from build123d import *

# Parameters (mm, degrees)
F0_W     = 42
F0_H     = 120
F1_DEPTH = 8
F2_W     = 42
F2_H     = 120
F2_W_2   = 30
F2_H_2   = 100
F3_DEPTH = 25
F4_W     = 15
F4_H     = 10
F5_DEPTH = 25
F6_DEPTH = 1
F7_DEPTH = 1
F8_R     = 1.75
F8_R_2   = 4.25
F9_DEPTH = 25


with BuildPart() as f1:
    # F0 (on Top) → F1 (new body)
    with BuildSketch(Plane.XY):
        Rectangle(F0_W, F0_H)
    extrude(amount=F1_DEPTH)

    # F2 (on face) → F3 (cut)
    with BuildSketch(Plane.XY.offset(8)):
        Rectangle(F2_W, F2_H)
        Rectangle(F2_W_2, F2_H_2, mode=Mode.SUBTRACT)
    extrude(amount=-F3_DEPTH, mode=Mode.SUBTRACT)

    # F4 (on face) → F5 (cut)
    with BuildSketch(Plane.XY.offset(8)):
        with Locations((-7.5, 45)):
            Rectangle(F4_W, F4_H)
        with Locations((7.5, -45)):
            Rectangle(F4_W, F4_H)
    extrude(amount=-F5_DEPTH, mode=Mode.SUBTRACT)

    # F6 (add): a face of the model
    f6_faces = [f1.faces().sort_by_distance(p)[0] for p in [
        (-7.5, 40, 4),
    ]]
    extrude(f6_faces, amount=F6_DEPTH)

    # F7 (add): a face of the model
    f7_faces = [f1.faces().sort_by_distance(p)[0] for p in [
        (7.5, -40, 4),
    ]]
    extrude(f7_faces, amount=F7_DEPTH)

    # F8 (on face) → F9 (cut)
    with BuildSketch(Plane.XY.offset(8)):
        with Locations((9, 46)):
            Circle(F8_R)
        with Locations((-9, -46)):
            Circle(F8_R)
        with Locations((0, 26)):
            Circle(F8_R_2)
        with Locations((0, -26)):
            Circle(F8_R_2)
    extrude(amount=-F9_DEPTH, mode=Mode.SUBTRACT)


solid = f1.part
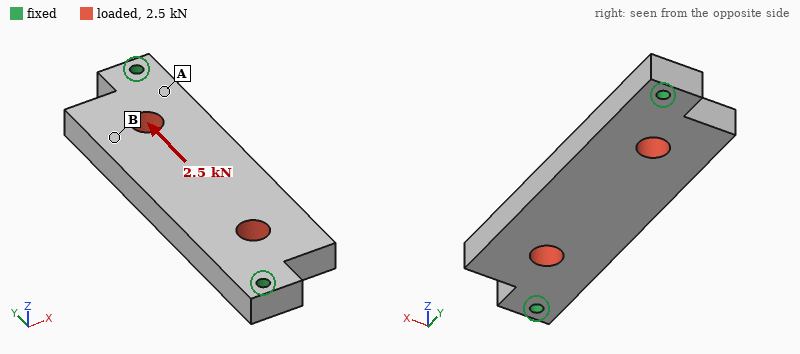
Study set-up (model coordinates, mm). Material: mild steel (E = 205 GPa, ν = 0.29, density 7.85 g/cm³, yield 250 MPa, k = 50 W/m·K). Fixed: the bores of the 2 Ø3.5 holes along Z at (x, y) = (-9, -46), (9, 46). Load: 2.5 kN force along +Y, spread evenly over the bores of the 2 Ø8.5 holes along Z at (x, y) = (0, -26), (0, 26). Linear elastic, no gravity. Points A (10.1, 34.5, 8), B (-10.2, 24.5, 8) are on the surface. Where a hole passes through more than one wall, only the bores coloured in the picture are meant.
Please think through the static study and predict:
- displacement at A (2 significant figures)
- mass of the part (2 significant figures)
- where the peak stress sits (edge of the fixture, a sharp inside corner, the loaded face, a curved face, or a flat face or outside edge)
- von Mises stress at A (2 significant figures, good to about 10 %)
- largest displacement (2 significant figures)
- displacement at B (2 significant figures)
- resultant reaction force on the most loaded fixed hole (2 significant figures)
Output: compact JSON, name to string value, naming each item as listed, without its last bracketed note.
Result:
{"displacement at A": "1.2 µm", "mass of the part": "160 g", "where the peak stress sits": "edge of the fixture", "von Mises stress at A": "11 MPa", "largest displacement": "3.3 µm", "displacement at B": "3.0 µm", "resultant reaction force on the most loaded fixed hole": "1.3 kN"}
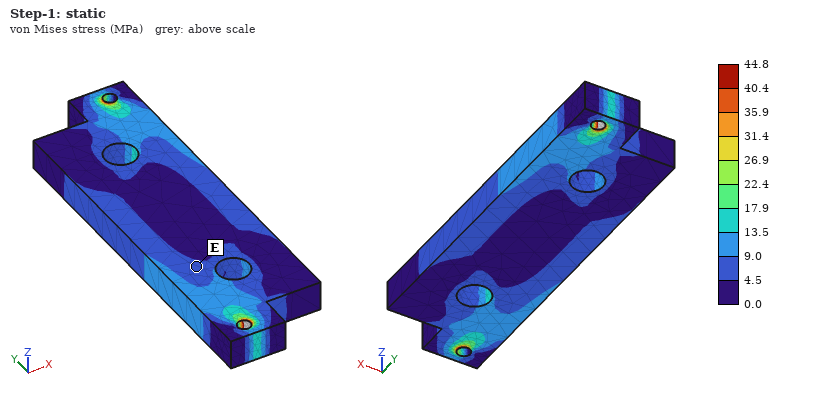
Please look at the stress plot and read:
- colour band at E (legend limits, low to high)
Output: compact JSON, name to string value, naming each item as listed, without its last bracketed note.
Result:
{"colour band at E": "4.5 to 9.0 MPa"}
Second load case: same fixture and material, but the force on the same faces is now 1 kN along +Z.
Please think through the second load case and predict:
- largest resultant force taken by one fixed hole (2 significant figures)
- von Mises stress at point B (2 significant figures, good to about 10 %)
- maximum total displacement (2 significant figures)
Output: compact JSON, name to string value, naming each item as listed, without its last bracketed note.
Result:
{"largest resultant force taken by one fixed hole": "500 N", "von Mises stress at point B": "13 MPa", "maximum total displacement": "13 µm"}
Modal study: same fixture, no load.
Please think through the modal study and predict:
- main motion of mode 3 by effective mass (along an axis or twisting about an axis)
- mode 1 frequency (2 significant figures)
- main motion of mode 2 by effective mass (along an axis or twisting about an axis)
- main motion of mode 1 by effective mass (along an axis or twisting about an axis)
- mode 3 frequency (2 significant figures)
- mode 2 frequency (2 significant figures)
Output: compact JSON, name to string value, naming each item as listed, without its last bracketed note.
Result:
{"main motion of mode 3 by effective mass": "along X", "mode 1 frequency": "3600 Hz", "main motion of mode 2 by effective mass": "twisting about Y", "main motion of mode 1 by effective mass": "along Z", "mode 3 frequency": "7100 Hz", "mode 2 frequency": "5300 Hz"}
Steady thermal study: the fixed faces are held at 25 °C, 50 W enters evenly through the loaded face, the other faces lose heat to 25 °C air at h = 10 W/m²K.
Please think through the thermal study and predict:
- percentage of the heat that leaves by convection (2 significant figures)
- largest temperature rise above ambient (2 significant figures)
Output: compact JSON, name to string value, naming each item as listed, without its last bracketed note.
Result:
{"percentage of the heat that leaves by convection": "8.0 %", "largest temperature rise above ambient": "79 K"}
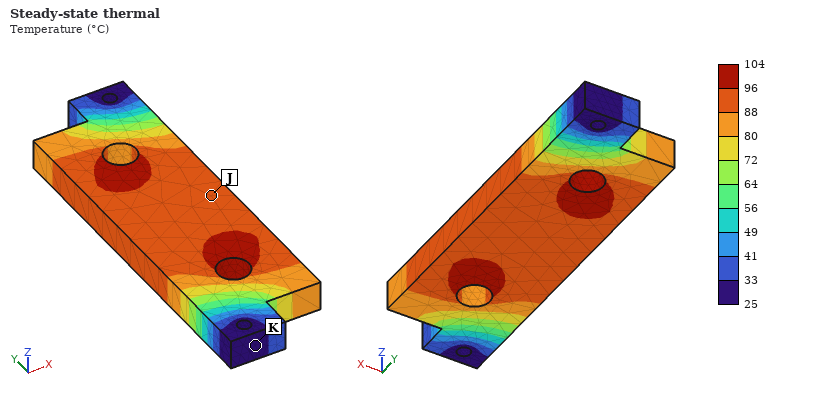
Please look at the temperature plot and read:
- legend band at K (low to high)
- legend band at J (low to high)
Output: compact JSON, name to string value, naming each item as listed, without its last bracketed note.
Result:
{"legend band at K": "25 to 33 °C", "legend band at J": "88 to 96 °C"}
